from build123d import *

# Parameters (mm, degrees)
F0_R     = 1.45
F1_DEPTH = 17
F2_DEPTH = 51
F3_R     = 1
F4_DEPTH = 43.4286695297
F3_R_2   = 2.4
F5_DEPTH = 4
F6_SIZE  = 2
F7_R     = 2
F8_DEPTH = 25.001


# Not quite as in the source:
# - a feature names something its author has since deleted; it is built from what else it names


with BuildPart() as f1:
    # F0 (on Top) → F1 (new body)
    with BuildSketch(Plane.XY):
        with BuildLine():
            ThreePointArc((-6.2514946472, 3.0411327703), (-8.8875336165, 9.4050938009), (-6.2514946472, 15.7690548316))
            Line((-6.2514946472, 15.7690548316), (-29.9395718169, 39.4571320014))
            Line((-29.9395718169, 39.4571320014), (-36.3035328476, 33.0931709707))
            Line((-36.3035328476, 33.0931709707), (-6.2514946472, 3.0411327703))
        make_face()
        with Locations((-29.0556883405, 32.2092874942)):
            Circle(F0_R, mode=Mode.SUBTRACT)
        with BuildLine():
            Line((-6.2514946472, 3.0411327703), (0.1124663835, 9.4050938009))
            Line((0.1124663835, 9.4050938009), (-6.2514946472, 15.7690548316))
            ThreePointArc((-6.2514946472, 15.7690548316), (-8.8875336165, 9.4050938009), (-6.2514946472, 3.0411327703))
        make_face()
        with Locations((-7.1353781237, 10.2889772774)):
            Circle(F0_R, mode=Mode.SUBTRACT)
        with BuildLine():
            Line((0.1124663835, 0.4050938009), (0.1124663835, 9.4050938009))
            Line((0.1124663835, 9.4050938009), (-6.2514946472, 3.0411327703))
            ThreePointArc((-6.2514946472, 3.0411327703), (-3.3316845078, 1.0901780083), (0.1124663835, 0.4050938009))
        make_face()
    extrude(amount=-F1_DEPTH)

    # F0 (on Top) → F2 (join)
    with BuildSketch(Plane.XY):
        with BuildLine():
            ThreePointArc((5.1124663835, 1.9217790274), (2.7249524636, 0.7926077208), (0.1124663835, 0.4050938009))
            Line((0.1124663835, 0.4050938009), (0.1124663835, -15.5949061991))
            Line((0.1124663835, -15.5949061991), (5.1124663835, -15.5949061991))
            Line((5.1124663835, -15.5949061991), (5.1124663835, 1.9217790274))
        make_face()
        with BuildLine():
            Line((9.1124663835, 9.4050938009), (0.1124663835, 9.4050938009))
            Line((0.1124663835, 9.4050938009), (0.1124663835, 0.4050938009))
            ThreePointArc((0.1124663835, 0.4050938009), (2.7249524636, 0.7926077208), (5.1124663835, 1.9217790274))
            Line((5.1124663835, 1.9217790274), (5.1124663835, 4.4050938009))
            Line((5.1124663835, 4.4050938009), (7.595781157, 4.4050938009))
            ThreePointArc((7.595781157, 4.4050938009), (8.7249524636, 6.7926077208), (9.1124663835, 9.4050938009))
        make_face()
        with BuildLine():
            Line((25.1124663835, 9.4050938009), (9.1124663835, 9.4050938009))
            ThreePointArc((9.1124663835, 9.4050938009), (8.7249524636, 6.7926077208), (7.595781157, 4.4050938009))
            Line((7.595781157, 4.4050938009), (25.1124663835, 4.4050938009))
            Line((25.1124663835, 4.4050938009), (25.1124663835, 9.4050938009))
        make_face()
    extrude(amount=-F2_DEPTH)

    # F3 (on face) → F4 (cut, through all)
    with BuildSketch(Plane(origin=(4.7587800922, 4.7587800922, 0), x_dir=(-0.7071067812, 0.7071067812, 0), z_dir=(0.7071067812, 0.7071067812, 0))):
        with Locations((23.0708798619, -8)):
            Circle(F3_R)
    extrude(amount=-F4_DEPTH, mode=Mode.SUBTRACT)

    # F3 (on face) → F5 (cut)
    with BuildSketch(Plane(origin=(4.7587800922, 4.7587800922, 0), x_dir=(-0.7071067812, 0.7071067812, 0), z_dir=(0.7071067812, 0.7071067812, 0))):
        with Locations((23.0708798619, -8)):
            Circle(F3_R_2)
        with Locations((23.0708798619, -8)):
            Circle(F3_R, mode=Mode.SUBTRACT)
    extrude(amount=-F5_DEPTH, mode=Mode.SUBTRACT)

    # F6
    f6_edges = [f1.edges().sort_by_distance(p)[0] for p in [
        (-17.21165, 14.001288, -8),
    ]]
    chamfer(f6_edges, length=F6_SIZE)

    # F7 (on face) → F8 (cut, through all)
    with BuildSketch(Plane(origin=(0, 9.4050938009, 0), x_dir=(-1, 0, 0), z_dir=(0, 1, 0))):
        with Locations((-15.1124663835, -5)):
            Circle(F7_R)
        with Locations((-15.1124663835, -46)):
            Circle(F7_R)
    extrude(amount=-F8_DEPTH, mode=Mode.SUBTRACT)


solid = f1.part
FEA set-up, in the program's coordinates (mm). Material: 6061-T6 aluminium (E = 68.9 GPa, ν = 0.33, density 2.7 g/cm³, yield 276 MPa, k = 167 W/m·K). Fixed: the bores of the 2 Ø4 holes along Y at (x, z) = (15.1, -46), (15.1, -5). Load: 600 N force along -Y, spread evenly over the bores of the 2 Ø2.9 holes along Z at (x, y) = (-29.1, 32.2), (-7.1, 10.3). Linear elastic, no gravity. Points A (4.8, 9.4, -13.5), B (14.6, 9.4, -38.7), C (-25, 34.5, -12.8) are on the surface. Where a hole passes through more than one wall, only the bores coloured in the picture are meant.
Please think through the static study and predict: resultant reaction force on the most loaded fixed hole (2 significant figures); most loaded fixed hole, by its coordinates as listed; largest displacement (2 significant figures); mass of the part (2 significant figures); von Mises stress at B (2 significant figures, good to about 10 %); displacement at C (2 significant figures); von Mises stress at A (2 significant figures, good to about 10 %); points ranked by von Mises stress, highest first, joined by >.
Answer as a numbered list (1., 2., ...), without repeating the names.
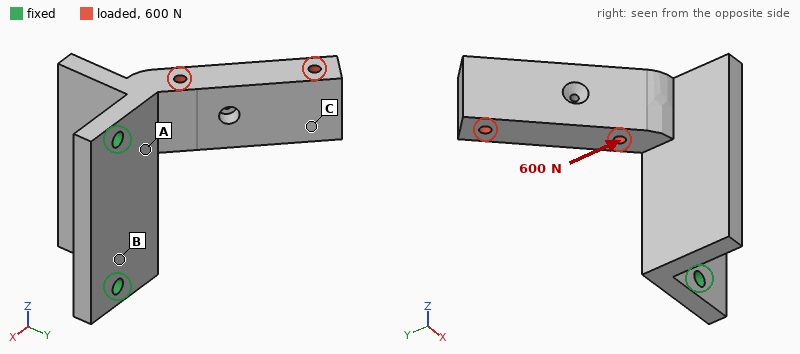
1. 540 N
2. (15.1, -5)
3. 0.59 mm
4. 49 g
5. 39 MPa
6. 0.48 mm
7. 91 MPa
8. A > B > C
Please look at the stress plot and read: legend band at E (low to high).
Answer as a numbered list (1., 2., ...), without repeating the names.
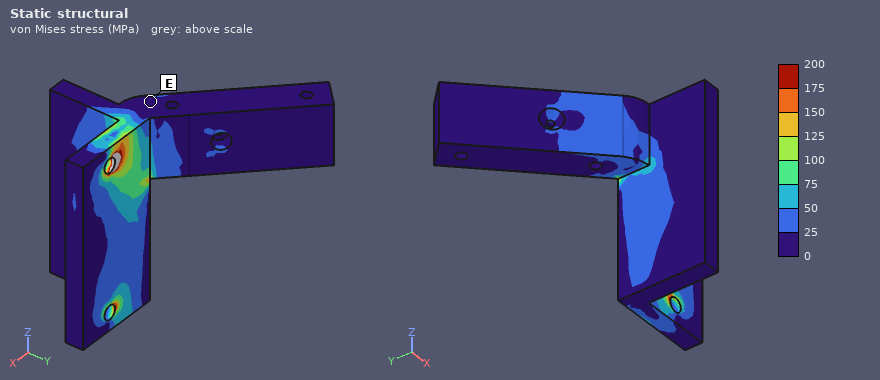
1. 0 to 25 MPa
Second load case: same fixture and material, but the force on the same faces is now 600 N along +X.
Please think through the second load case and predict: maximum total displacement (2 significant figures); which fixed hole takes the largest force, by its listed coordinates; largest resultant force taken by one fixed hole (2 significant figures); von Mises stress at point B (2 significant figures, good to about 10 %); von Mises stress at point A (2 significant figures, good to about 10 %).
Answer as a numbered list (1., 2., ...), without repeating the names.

1. 0.35 mm
2. (15.1, -5)
3. 550 N
4. 20 MPa
5. 61 MPa
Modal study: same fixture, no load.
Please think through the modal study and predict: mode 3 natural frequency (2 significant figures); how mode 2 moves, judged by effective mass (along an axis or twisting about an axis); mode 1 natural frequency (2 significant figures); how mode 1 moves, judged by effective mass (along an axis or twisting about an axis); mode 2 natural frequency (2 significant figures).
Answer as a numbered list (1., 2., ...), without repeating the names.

1. 5500 Hz
2. along Z
3. 1400 Hz
4. along Y
5. 3500 Hz
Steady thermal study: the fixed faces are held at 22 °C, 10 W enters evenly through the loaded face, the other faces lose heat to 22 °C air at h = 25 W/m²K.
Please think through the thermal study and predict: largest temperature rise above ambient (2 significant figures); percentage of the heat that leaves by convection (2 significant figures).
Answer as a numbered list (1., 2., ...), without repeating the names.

1. 16 K
2. 11 %
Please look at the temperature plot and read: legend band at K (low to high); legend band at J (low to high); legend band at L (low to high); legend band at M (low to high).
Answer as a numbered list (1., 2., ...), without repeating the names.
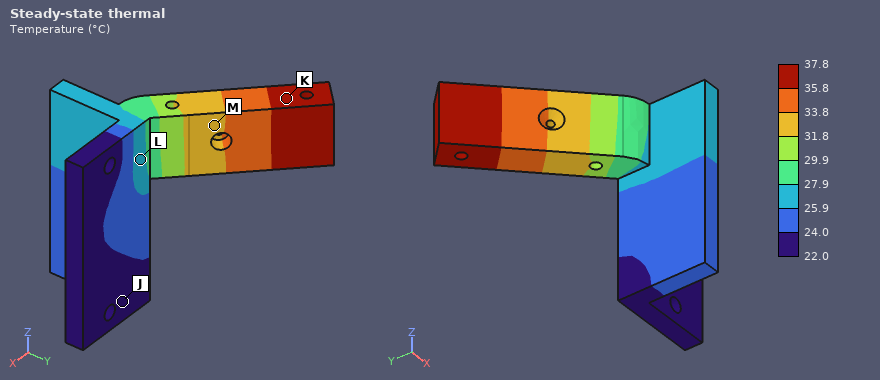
1. 35.8 to 37.8 °C
2. 22.0 to 24.0 °C
3. 25.9 to 27.9 °C
4. 31.8 to 33.8 °C
